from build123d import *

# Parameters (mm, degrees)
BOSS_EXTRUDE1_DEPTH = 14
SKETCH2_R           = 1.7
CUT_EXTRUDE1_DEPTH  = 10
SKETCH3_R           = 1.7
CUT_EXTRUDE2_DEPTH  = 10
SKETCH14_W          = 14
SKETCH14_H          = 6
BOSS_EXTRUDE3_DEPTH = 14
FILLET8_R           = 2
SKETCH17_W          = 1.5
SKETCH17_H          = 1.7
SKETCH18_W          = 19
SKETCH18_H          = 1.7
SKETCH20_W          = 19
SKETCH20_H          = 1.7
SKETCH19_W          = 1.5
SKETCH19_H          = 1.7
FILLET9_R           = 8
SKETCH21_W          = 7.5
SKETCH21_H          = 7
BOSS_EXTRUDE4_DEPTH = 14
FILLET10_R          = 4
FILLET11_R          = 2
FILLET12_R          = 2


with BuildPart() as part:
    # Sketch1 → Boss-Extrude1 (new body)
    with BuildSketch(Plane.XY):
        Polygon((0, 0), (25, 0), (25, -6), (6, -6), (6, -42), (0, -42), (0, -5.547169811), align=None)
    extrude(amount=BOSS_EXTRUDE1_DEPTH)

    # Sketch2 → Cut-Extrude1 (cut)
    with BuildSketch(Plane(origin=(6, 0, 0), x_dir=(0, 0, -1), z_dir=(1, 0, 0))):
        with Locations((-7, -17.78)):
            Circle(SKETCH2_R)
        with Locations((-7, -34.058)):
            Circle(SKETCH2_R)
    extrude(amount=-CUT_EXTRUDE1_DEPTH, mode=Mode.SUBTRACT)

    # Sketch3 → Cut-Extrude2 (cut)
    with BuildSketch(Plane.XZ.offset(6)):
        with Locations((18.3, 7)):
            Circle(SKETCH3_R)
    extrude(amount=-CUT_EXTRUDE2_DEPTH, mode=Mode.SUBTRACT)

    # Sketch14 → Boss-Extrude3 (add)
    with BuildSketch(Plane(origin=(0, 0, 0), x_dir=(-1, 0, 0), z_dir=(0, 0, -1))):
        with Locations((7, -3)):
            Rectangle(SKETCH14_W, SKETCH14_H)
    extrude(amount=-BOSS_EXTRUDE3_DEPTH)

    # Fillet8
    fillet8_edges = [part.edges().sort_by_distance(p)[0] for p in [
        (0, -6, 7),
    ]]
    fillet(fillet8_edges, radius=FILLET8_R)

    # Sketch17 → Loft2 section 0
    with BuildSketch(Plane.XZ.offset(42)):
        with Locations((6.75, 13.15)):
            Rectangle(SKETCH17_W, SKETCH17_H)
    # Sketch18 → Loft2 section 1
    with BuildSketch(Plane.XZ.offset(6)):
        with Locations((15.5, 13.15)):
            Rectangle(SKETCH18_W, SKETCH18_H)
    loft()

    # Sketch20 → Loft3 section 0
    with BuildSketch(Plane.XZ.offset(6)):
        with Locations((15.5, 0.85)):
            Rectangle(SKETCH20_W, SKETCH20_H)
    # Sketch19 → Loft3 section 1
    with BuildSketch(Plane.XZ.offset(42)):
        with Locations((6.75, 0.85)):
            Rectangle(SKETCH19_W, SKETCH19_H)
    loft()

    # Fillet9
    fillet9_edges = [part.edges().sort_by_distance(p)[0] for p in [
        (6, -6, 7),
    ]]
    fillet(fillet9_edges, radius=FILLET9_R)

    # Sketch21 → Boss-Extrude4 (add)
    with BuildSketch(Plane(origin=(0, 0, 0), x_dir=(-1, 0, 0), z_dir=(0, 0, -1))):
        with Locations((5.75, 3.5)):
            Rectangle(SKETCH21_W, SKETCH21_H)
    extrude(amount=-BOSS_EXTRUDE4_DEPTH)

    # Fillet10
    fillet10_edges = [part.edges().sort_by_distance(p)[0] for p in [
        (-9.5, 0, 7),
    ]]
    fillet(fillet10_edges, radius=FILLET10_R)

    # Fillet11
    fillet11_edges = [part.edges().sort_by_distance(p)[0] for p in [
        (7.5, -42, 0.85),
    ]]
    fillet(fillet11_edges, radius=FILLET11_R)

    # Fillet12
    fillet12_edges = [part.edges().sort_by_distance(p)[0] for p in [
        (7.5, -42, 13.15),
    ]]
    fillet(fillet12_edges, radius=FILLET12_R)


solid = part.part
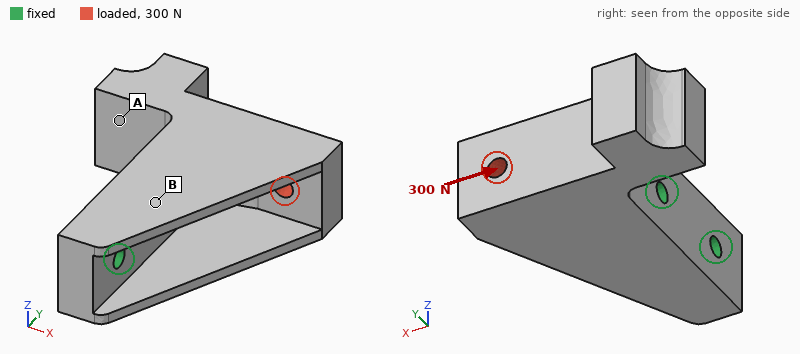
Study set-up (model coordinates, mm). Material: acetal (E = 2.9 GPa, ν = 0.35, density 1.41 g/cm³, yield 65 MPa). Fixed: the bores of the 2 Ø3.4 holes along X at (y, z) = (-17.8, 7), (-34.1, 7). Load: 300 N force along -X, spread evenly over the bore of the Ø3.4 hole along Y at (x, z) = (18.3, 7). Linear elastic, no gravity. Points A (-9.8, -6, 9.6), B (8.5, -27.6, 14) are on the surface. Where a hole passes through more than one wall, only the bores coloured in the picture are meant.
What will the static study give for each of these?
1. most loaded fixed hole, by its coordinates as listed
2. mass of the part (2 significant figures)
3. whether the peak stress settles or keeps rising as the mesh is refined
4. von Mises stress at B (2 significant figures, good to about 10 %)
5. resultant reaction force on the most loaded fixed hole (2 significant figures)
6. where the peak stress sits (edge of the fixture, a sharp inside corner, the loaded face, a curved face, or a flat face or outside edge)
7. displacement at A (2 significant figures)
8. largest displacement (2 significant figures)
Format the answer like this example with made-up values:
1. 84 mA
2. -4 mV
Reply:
1. (-17.8, 7)
2. 12 g
3. keeps rising
4. 5.9 MPa
5. 460 N
6. edge of the fixture
7. 0.19 mm
8. 0.30 mm
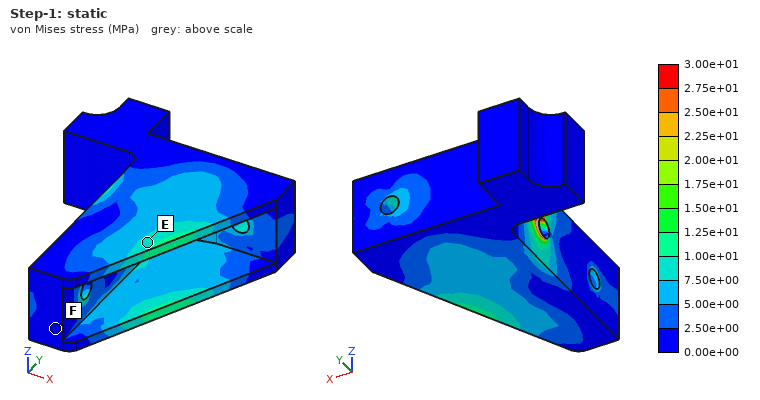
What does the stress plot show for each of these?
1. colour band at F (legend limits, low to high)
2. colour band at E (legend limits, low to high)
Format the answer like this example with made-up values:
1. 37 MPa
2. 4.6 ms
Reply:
1. 0.00e+00 to 2.50e+00 MPa
2. 7.50e+00 to 1.00e+01 MPa
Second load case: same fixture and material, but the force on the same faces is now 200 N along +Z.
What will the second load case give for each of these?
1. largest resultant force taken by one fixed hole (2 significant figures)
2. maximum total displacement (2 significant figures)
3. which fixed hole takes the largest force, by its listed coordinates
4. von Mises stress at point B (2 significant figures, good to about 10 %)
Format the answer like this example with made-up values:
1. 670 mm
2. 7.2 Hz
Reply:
1. 320 N
2. 0.67 mm
3. (-17.8, 7)
4. 5.6 MPa
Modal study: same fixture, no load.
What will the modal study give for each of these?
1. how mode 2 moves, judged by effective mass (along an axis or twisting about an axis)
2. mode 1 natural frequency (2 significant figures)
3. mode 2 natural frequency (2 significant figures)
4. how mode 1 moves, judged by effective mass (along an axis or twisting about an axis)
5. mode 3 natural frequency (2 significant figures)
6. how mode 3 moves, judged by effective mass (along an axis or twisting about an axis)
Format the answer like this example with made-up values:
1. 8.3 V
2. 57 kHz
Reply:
1. along X
2. 1800 Hz
3. 2000 Hz
4. twisting about Y
5. 2300 Hz
6. along Z
